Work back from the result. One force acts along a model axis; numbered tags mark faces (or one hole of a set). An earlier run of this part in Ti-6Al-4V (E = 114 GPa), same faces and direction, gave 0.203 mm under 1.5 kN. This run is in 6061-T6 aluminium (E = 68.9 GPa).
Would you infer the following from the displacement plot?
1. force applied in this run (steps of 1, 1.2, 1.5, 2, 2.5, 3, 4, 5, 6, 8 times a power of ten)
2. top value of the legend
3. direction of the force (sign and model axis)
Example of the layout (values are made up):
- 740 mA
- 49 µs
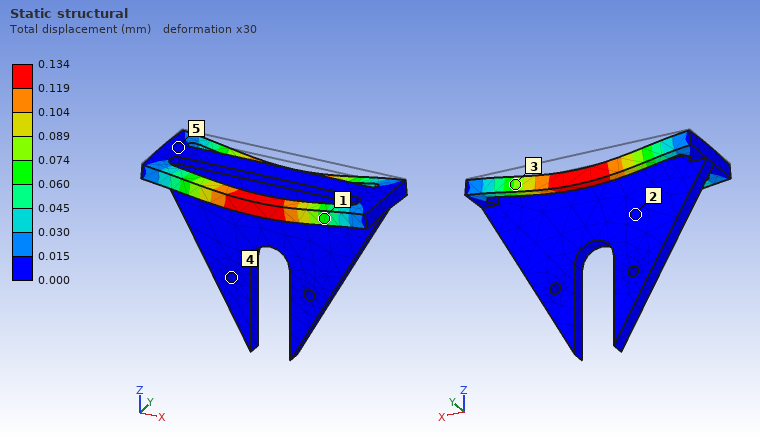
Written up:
- 600 N
- 0.134 mm
- -Z
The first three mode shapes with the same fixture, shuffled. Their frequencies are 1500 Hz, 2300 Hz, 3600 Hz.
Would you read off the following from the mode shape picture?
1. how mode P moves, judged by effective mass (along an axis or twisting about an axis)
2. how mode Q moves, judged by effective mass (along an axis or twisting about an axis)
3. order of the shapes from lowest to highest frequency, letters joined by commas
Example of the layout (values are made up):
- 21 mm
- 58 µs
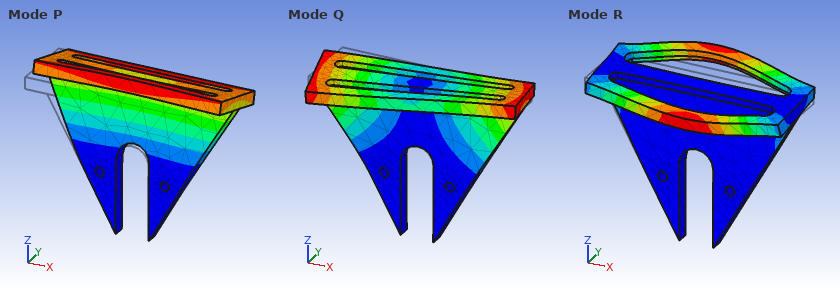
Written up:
- along Y
- twisting about Z
- P, Q, R
